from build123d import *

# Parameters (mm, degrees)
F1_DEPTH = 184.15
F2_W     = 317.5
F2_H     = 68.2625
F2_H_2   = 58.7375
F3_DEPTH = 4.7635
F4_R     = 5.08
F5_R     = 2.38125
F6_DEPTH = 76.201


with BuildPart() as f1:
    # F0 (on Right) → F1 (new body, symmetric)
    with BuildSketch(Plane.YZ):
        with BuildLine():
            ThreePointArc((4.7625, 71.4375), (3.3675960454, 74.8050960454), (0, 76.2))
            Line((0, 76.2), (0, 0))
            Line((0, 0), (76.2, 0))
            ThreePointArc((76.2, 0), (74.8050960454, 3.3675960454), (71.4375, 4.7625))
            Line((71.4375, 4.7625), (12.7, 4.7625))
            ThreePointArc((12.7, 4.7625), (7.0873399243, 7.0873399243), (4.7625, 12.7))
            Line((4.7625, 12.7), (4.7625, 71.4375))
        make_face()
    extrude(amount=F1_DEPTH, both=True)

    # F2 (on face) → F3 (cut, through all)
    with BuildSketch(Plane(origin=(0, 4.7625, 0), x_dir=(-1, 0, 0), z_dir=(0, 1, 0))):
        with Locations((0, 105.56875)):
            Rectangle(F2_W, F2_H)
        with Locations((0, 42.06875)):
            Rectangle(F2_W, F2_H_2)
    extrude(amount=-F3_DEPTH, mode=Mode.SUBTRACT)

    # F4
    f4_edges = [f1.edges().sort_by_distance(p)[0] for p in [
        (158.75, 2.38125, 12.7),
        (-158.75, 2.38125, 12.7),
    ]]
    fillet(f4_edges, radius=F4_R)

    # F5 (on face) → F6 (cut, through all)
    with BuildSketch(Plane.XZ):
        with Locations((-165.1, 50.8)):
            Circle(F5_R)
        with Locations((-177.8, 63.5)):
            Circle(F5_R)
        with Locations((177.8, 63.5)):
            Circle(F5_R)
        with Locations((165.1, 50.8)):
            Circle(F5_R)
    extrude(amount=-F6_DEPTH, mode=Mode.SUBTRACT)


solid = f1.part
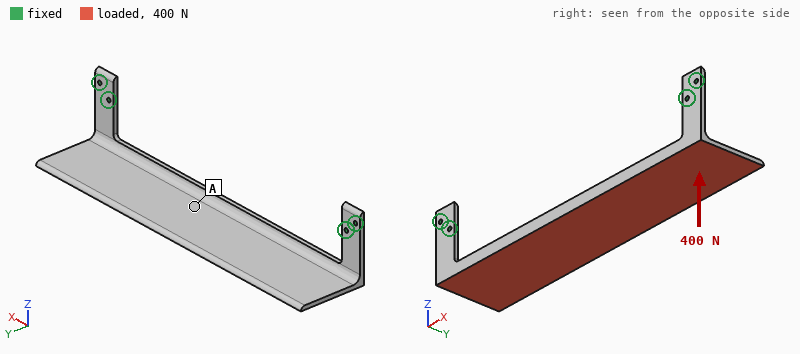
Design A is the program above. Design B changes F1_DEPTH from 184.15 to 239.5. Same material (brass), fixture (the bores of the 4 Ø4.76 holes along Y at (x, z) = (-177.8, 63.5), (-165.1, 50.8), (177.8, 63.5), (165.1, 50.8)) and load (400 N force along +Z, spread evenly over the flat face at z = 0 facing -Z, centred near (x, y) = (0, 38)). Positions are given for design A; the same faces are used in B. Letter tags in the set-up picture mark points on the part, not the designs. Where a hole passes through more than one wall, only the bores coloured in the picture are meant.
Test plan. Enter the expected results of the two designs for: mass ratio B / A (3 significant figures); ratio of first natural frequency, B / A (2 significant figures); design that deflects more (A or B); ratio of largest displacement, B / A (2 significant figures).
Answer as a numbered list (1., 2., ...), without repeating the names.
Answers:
1. 1.47
2. 1.2
3. A
4. 0.54
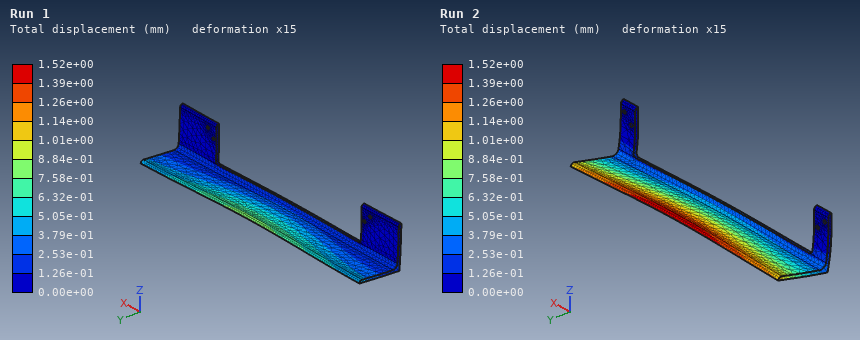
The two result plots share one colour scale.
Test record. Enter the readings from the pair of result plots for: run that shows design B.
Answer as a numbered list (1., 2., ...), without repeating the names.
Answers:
1. Run 1
